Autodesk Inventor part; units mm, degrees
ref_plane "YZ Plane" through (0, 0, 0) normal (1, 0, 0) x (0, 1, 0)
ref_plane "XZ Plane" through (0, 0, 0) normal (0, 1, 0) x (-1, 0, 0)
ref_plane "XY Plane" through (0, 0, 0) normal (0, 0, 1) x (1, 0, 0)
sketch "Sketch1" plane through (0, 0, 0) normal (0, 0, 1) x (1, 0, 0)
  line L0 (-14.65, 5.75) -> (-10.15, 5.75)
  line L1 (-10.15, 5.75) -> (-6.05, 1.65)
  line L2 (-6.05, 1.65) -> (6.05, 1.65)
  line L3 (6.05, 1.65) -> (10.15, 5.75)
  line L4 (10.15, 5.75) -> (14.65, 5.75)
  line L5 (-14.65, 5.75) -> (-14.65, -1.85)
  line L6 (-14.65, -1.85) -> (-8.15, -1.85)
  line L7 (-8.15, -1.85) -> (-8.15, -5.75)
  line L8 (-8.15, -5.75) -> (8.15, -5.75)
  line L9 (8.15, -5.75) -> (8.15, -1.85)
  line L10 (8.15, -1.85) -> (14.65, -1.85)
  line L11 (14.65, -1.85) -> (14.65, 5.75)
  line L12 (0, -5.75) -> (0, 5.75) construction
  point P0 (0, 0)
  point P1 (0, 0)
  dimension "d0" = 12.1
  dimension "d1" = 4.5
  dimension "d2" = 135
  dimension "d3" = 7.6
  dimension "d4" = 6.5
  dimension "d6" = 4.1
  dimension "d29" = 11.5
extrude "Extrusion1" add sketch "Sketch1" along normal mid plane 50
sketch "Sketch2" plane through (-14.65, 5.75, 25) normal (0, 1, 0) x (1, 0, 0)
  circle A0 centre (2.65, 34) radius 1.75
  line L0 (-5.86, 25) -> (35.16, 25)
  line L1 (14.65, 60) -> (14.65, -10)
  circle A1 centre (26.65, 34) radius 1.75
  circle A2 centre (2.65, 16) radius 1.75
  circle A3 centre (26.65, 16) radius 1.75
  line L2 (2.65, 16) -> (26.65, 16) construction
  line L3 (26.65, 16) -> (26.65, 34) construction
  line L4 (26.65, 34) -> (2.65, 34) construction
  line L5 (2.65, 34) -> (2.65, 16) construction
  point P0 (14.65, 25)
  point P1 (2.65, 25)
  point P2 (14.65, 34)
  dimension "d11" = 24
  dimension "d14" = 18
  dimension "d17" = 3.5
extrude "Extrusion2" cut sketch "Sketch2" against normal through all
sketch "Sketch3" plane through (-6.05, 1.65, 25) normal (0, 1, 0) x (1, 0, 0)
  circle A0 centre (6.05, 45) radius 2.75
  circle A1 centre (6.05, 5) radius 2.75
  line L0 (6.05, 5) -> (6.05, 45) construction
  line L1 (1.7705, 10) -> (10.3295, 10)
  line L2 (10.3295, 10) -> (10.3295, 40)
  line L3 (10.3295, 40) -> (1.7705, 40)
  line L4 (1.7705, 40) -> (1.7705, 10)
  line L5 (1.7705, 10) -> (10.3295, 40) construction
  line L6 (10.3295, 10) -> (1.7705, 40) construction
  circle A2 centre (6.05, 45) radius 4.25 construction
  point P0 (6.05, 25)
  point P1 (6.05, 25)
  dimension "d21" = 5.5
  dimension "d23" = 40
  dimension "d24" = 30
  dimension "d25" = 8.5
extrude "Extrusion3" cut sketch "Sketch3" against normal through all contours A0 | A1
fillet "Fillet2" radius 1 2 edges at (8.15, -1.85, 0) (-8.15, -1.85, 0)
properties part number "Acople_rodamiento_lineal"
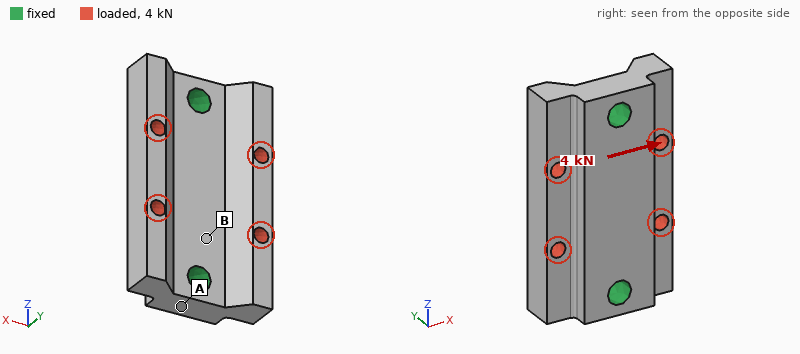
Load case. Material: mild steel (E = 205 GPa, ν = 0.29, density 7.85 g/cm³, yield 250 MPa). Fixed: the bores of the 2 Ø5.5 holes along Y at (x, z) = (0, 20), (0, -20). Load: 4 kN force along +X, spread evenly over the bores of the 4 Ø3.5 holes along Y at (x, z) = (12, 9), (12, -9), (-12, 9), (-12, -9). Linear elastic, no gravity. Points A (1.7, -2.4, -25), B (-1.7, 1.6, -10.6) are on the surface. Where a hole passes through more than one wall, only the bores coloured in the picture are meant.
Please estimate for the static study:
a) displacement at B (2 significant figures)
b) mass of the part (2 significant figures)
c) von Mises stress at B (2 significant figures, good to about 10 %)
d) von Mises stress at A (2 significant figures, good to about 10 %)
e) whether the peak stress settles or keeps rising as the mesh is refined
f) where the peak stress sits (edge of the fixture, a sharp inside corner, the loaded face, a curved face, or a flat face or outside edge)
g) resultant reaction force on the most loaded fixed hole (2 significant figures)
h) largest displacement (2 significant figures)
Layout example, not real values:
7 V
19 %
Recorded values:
3.2 µm
81 g
38 MPa
16 MPa
keeps rising
edge of the fixture
2.0 kN
11 µm
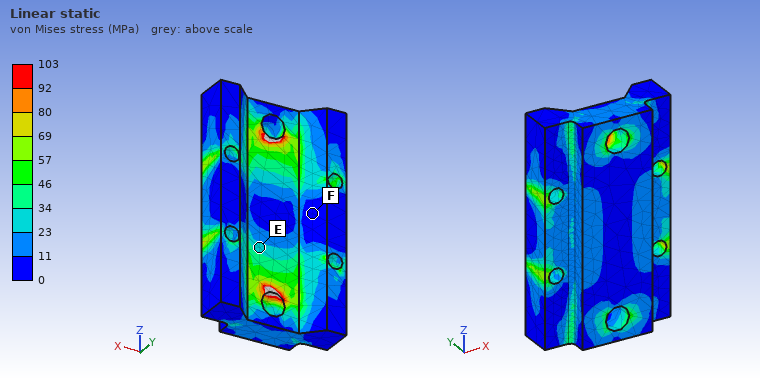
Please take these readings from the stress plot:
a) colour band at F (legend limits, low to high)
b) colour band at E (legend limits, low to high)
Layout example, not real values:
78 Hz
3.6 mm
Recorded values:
0 to 11 MPa
23 to 34 MPa
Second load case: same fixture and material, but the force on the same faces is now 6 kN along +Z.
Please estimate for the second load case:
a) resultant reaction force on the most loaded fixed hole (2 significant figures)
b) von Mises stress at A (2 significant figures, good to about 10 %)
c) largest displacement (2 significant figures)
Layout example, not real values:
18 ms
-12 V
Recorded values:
3.1 kN
26 MPa
2.9 µm
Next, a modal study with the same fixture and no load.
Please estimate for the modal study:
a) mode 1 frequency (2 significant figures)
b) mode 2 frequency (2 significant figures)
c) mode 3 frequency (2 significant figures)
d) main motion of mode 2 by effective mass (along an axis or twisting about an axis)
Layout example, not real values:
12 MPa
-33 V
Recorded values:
14 kHz
17 kHz
24 kHz
along Y
